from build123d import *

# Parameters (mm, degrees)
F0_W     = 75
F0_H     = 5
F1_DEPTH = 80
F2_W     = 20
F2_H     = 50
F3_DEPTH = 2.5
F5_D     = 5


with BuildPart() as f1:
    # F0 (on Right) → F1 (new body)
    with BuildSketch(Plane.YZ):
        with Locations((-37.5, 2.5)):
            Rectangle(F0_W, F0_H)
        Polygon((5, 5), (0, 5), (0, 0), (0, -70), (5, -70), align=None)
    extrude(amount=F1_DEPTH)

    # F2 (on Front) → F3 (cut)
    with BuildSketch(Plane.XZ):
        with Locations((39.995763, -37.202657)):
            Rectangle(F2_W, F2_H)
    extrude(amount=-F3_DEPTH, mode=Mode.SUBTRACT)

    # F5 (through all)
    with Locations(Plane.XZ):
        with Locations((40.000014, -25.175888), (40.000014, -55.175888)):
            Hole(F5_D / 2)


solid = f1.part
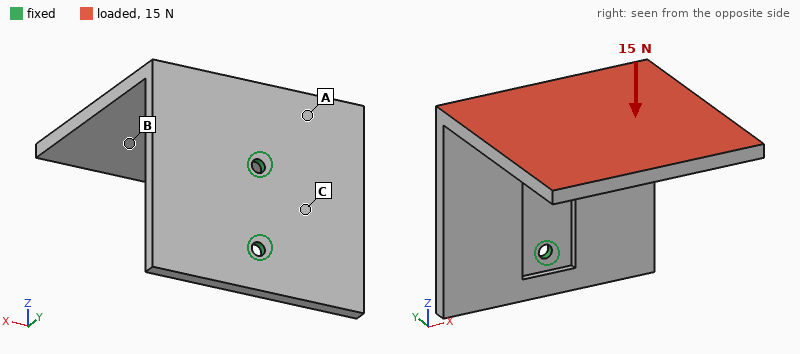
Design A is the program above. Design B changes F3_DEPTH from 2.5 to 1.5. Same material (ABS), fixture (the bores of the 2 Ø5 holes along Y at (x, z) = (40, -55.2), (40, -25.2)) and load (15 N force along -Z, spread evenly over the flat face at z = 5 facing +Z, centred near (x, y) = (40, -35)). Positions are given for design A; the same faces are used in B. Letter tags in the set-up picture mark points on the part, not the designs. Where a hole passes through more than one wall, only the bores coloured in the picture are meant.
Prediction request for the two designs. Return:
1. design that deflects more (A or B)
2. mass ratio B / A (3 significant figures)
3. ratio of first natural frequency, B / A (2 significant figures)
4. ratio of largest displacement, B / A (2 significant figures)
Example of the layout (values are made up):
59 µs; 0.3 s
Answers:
A; 1.02; 1.1; 0.89
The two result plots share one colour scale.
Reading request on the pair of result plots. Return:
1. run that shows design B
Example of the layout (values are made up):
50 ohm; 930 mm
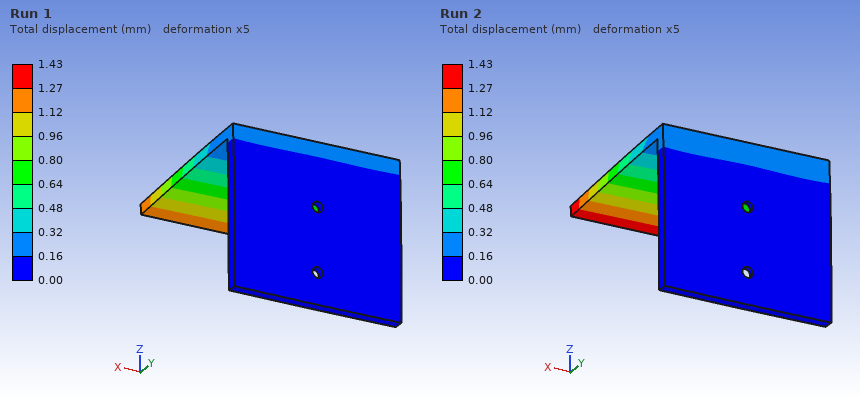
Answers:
Run 1
